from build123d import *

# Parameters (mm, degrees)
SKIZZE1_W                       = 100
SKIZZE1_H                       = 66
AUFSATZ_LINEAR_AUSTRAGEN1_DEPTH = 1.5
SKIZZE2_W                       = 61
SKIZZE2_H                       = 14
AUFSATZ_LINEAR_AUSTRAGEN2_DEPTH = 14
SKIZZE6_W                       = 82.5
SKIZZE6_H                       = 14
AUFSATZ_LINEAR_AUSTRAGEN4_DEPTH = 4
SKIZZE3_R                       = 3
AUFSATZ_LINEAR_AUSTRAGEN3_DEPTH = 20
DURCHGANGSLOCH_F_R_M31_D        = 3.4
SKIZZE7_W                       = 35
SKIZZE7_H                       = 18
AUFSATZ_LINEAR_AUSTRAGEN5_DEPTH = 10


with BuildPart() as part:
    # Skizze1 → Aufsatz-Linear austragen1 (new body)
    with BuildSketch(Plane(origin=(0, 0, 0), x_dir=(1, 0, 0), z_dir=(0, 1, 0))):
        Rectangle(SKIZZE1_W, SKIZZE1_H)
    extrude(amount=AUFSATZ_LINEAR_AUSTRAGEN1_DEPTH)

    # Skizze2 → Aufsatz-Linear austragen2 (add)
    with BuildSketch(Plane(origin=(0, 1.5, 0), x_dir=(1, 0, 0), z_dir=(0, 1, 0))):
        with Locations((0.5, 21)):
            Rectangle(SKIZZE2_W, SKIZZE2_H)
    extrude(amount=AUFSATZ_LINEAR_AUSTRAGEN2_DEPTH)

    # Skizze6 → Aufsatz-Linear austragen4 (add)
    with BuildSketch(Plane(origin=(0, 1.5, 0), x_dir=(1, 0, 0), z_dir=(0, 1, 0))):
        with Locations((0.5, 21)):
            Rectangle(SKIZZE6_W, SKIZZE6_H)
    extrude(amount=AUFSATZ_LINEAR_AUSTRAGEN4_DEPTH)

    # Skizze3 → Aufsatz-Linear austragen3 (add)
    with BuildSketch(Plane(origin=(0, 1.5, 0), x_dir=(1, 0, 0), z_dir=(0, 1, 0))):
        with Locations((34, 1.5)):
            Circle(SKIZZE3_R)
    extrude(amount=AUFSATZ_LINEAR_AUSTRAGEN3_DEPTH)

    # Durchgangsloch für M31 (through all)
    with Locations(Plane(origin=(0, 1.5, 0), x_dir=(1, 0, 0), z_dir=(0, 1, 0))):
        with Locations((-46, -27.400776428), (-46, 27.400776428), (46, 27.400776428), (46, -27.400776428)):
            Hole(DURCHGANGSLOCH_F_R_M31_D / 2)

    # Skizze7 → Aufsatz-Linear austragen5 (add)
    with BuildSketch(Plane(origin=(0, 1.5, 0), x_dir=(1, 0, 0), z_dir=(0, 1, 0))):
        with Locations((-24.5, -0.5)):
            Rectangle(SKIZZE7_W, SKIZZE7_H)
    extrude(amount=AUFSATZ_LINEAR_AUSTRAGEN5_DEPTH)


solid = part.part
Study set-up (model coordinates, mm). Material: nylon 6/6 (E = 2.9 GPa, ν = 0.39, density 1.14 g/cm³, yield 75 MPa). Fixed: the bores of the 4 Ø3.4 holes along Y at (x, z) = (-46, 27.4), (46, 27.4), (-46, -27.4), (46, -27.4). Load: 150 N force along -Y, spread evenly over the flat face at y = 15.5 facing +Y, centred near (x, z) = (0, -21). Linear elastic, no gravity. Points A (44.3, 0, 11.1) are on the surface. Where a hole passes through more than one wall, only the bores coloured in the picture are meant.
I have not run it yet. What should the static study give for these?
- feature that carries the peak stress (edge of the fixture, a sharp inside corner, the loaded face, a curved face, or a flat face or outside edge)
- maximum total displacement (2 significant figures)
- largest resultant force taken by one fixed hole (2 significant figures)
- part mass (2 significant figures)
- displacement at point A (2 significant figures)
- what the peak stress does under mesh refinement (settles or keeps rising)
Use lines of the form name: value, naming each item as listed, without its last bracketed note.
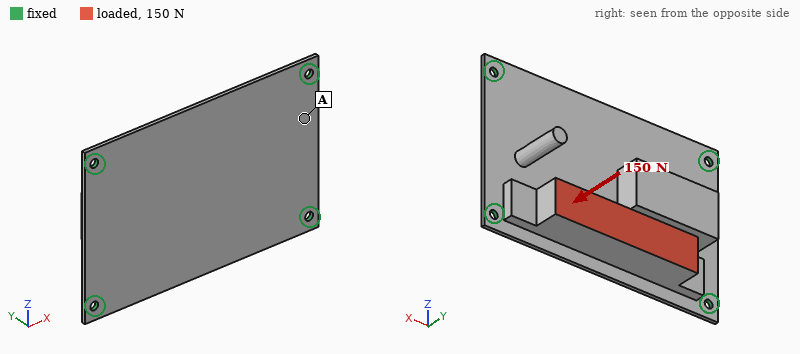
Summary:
feature that carries the peak stress: edge of the fixture
maximum total displacement: 0.62 mm
largest resultant force taken by one fixed hole: 130 N
part mass: 34 g
displacement at point A: 0.24 mm
what the peak stress does under mesh refinement: keeps rising
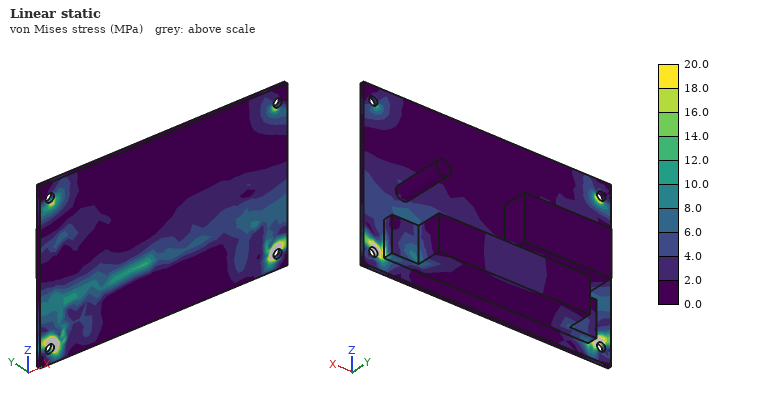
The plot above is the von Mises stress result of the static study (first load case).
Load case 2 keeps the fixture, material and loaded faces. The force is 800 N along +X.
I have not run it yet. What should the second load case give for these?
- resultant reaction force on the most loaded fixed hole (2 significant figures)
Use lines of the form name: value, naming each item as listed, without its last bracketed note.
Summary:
resultant reaction force on the most loaded fixed hole: 370 N
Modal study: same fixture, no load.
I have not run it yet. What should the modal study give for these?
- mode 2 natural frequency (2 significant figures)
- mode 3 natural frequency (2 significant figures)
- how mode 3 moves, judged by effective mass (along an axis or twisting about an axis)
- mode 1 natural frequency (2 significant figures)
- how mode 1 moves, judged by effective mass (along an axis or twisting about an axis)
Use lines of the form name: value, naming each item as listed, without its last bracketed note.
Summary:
mode 2 natural frequency: 630 Hz
mode 3 natural frequency: 840 Hz
how mode 3 moves, judged by effective mass: twisting about Z
mode 1 natural frequency: 350 Hz
how mode 1 moves, judged by effective mass: along Y
